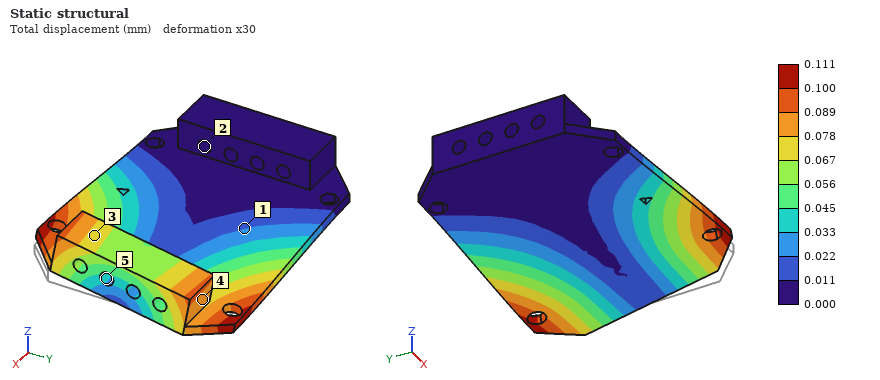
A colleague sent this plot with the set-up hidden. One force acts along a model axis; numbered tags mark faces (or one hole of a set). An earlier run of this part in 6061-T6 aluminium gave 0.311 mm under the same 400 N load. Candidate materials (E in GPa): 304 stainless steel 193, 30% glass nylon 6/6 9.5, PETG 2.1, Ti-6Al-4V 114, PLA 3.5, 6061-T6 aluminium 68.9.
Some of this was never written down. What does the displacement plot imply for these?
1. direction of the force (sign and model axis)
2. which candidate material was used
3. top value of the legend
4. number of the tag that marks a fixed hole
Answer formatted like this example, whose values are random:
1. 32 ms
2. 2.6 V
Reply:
1. +Y
2. 304 stainless steel
3. 0.111 mm
4. 2
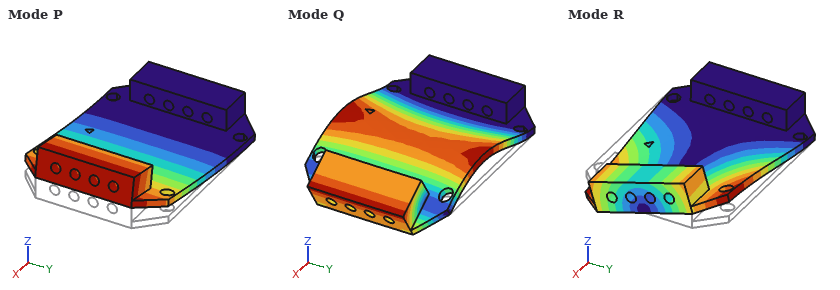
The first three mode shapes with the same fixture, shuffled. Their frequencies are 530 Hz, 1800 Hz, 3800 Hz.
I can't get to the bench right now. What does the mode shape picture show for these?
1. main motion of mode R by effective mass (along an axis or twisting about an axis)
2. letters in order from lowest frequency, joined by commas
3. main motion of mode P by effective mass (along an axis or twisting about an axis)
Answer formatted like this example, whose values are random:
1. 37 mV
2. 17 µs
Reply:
1. twisting about X
2. P, R, Q
3. along Z
